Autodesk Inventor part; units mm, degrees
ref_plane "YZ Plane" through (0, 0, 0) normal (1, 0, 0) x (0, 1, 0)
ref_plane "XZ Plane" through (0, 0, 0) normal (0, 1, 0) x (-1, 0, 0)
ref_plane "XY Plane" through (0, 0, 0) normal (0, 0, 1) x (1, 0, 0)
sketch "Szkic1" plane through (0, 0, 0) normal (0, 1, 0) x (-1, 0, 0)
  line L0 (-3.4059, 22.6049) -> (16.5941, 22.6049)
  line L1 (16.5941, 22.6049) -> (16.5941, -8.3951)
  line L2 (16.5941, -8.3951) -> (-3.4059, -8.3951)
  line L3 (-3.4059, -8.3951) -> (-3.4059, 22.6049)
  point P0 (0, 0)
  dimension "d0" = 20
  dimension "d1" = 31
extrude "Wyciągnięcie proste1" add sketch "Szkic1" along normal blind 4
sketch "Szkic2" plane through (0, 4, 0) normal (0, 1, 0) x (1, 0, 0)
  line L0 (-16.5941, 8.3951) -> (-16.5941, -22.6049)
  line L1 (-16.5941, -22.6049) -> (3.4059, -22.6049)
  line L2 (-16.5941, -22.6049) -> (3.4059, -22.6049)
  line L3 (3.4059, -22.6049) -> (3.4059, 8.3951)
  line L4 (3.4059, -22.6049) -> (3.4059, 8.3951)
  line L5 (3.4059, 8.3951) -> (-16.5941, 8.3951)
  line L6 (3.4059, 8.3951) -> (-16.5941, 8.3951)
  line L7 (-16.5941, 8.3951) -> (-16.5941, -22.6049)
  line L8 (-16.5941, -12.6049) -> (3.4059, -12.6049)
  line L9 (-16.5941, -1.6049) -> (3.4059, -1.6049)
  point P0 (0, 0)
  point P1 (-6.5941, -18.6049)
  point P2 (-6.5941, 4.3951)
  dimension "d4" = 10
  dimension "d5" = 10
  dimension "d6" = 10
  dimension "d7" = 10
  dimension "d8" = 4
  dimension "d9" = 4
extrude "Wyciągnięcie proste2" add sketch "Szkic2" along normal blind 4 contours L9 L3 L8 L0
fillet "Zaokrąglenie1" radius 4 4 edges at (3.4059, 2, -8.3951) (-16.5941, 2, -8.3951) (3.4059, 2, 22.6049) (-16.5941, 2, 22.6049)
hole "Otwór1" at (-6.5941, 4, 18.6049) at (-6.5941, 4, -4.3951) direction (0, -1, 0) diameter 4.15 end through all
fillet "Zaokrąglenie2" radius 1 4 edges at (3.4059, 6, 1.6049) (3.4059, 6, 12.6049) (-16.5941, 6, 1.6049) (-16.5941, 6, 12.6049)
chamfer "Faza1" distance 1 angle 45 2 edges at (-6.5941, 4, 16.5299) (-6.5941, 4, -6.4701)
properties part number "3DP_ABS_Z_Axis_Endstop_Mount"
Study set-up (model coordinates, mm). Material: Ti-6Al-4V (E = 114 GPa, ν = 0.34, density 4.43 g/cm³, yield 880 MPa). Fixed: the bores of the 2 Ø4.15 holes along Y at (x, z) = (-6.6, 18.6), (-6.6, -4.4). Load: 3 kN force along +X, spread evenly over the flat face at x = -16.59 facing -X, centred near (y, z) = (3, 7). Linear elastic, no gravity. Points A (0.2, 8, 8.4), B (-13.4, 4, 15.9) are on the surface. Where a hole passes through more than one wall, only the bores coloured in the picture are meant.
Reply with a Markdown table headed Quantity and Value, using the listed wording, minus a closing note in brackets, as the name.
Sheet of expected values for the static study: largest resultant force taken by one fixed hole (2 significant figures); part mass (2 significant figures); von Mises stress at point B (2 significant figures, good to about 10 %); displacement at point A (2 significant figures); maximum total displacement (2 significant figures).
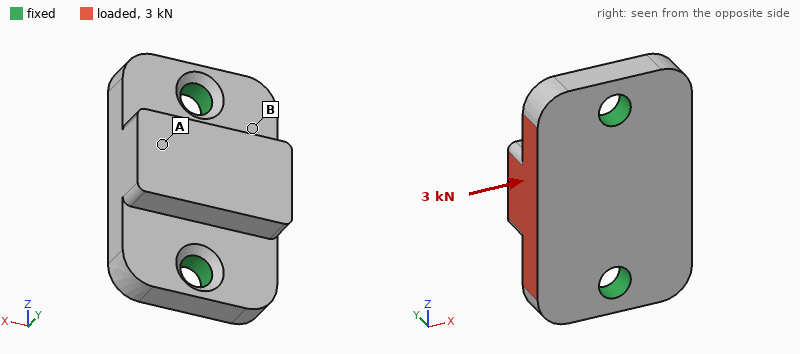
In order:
| Quantity | Value |
|---|---|
| largest resultant force taken by one fixed hole | 1.5 kN |
| part mass | 14 g |
| von Mises stress at point B | 39 MPa |
| displacement at point A | 11 µm |
| maximum total displacement | 16 µm |
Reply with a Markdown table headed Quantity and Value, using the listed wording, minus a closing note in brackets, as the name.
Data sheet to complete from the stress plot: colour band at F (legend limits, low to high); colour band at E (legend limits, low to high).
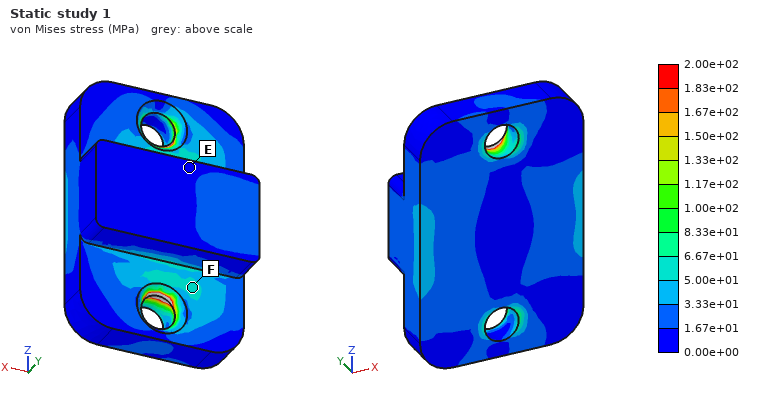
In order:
| Quantity | Value |
|---|---|
| colour band at F | 5.00e+01 to 6.67e+01 MPa |
| colour band at E | 0.00e+00 to 1.67e+01 MPa |
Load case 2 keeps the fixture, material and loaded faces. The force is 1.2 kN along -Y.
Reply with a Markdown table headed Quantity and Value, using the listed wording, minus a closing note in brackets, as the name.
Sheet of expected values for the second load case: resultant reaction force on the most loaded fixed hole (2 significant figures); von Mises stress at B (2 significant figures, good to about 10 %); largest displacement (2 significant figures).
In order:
| Quantity | Value |
|---|---|
| resultant reaction force on the most loaded fixed hole | 690 N |
| von Mises stress at B | 38 MPa |
| largest displacement | 36 µm |
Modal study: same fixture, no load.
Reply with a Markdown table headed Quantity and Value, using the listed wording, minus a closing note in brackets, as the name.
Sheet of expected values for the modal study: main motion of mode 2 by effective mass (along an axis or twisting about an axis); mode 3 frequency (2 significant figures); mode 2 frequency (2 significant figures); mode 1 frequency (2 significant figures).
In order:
| Quantity | Value |
|---|---|
| main motion of mode 2 by effective mass | along Y |
| mode 3 frequency | 41 kHz |
| mode 2 frequency | 25 kHz |
| mode 1 frequency | 16 kHz |
